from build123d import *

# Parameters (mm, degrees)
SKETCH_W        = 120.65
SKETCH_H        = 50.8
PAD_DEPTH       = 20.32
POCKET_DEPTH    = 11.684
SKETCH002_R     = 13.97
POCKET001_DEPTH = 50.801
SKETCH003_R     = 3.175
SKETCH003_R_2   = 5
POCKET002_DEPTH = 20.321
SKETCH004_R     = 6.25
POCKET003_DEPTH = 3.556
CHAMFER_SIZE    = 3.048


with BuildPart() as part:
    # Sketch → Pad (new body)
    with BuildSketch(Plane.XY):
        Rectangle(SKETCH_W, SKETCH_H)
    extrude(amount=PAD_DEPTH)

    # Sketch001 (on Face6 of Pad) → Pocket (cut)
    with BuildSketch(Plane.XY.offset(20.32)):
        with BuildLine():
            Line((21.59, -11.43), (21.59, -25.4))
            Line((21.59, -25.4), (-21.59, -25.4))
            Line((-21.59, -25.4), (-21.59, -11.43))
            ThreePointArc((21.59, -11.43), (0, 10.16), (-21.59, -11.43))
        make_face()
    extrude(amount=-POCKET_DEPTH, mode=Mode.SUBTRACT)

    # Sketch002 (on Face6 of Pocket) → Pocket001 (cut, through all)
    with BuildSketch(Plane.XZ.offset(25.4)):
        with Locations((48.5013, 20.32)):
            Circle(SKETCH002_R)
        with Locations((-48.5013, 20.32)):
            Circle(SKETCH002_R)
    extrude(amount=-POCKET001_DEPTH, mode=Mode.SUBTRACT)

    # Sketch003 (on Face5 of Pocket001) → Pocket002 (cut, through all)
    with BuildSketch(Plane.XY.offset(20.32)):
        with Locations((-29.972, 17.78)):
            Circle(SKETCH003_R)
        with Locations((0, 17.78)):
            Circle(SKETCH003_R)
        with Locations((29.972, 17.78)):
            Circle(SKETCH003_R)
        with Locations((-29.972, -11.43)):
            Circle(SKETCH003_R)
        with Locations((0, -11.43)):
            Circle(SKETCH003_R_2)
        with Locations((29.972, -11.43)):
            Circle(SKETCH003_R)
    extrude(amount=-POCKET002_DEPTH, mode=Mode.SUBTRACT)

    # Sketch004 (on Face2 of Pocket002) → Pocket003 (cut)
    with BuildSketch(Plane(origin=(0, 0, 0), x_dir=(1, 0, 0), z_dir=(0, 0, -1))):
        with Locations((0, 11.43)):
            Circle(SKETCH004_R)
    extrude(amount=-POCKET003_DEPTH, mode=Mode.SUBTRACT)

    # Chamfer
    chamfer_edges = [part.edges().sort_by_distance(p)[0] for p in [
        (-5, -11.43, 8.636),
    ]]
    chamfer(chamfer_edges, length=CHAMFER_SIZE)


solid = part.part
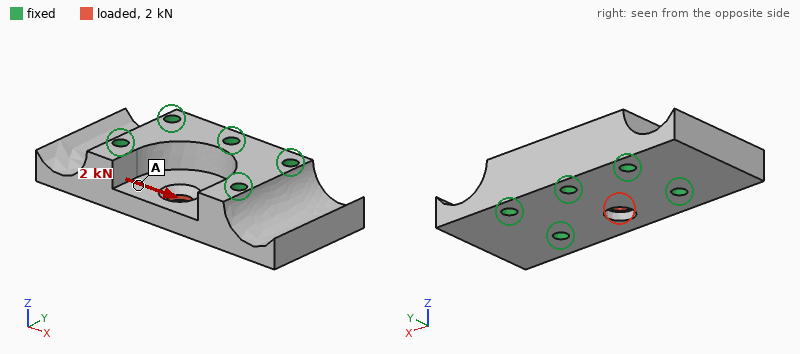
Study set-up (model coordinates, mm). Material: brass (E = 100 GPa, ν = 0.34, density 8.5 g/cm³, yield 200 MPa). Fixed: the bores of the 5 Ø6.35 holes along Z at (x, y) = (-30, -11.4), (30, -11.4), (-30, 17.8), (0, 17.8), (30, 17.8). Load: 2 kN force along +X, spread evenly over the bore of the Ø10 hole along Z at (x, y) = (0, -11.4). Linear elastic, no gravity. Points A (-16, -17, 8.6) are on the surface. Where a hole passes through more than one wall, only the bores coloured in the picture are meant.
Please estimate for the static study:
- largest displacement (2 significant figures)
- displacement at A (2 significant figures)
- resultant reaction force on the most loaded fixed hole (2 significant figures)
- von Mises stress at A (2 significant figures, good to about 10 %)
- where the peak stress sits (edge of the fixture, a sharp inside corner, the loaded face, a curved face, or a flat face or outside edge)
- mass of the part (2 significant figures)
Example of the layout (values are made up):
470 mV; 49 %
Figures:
2.3 µm; 0.67 µm; 770 N; 5.7 MPa; a sharp inside corner; 630 g
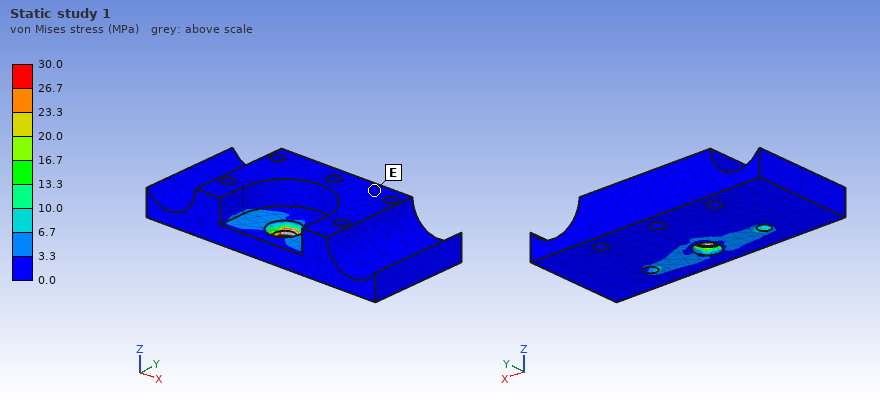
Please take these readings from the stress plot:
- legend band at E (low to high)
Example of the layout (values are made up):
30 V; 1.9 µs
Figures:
0.0 to 3.3 MPa
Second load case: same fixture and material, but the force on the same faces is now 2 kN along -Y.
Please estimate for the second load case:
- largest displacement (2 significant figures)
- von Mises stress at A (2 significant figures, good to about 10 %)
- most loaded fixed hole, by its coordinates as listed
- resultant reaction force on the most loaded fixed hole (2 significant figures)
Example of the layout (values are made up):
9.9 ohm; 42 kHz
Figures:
3.3 µm; 3.3 MPa; (0, 17.8); 850 N
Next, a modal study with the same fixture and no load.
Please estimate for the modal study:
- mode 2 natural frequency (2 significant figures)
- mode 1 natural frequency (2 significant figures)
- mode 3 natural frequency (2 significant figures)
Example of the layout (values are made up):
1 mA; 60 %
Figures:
6100 Hz; 6100 Hz; 8400 Hz
